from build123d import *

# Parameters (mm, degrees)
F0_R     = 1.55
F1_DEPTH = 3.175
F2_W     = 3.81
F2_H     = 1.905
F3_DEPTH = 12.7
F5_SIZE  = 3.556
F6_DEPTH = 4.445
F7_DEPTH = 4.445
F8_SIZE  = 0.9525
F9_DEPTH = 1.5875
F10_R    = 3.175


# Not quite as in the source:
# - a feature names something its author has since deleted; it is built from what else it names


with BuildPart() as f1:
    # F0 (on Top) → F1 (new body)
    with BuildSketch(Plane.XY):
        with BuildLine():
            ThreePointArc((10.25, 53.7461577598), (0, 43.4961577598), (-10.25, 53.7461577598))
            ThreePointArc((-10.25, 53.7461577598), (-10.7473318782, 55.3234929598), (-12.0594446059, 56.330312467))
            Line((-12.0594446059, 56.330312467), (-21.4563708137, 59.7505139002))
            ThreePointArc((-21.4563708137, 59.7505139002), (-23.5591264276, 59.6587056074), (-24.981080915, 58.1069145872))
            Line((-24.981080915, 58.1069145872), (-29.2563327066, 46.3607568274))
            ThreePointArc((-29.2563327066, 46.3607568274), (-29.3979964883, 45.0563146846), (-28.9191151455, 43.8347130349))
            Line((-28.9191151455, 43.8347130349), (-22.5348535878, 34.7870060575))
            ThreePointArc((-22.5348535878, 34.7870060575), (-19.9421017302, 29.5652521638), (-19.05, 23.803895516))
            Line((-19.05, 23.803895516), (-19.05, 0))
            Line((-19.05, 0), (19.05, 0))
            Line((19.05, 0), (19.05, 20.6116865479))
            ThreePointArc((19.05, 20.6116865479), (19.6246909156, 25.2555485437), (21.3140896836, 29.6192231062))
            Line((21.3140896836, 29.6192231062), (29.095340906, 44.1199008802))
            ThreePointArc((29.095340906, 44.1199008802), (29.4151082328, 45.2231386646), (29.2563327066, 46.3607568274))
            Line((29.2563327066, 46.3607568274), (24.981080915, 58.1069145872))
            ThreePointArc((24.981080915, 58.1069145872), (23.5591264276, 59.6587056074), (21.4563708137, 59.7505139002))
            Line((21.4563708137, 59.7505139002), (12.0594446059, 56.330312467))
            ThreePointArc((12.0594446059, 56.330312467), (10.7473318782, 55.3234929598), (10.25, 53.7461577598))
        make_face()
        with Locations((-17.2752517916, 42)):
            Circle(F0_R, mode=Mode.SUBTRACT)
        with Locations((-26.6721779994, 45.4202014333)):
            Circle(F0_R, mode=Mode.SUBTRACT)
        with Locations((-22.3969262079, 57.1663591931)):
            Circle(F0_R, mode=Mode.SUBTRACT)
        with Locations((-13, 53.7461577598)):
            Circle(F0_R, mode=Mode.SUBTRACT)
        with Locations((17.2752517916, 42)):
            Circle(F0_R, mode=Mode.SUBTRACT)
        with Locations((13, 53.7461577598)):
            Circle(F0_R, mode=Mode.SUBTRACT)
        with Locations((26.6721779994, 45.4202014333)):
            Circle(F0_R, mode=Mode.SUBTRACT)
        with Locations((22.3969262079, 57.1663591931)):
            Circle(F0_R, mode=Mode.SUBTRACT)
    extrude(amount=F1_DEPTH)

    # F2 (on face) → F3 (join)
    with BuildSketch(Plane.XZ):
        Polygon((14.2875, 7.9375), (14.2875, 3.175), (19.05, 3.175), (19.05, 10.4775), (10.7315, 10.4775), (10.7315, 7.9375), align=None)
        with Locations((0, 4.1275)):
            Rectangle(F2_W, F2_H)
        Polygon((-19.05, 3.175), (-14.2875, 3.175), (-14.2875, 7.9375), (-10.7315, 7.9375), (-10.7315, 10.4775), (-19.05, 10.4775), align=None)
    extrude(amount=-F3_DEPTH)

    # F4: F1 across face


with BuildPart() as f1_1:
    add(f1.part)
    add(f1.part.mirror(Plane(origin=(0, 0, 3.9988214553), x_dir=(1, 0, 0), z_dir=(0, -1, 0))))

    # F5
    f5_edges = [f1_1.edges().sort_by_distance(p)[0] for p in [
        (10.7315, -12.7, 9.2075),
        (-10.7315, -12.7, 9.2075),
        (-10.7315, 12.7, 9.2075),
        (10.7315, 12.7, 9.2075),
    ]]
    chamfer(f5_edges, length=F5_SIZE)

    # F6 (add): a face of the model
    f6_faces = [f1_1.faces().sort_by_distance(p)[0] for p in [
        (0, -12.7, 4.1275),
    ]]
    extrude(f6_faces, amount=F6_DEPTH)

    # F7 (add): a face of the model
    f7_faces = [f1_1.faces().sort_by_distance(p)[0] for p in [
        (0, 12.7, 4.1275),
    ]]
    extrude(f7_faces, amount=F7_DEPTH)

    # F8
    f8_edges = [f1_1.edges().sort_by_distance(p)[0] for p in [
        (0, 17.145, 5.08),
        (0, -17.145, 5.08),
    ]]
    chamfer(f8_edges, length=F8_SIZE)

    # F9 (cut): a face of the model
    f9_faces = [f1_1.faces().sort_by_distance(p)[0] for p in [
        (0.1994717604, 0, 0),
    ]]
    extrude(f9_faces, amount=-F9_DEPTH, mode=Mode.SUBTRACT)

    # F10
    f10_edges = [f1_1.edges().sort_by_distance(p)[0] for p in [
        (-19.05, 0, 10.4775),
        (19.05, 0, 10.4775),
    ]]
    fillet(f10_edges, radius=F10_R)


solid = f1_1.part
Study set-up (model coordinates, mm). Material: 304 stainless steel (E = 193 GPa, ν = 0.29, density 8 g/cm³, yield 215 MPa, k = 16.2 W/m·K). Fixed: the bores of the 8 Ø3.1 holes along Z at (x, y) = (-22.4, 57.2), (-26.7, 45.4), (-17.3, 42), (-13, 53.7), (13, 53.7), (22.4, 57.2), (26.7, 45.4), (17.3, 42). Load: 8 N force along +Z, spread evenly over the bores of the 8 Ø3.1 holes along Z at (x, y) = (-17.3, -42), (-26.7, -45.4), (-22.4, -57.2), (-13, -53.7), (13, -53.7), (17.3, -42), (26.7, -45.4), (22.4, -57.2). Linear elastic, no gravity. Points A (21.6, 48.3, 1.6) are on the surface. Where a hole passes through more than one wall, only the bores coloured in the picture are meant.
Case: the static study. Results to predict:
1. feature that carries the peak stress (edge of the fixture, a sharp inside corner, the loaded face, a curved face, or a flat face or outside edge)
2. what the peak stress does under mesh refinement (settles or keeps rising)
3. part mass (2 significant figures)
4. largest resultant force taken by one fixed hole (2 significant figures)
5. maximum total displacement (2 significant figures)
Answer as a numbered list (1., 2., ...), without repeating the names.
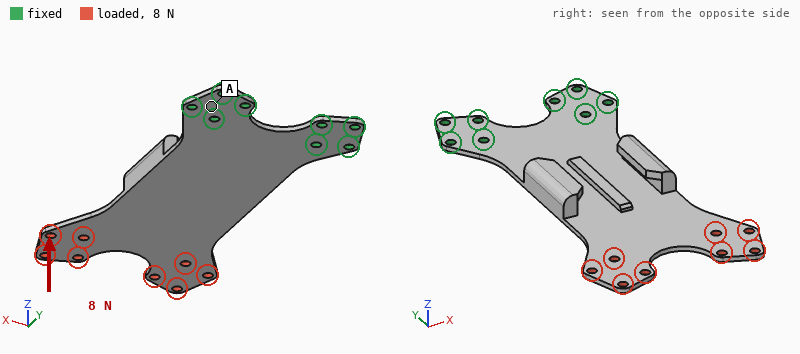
1. edge of the fixture
2. keeps rising
3. 77 g
4. 26 N
5. 0.71 mm
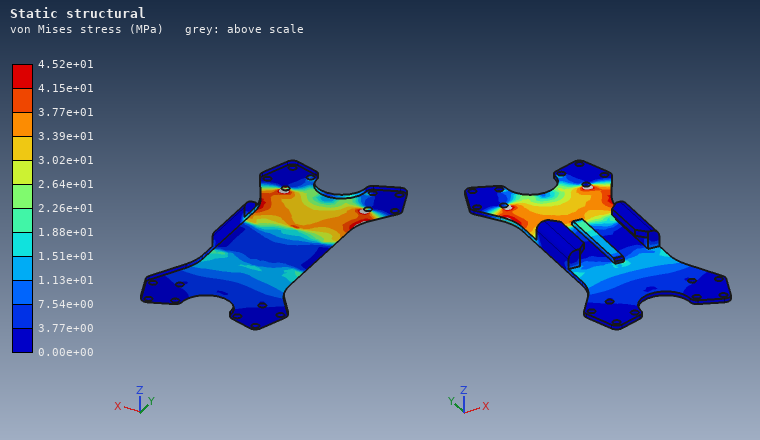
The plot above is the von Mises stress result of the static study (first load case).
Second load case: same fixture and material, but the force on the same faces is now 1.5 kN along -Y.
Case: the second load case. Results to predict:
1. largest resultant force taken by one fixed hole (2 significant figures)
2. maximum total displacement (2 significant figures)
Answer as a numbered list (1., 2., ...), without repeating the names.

1. 490 N
2. 61 µm
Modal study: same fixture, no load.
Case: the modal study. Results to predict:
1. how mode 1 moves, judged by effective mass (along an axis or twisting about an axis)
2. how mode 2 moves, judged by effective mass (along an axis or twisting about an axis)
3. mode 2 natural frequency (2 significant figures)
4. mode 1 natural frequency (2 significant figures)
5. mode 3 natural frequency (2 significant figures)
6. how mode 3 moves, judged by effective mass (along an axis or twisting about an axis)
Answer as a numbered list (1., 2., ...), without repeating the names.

1. along Z
2. twisting about Y
3. 580 Hz
4. 130 Hz
5. 880 Hz
6. along Z
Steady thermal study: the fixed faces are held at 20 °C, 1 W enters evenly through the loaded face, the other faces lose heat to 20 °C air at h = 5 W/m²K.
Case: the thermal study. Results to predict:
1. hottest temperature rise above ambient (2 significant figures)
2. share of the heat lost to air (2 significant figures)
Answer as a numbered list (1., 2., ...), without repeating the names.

1. 42 K
2. 76 %
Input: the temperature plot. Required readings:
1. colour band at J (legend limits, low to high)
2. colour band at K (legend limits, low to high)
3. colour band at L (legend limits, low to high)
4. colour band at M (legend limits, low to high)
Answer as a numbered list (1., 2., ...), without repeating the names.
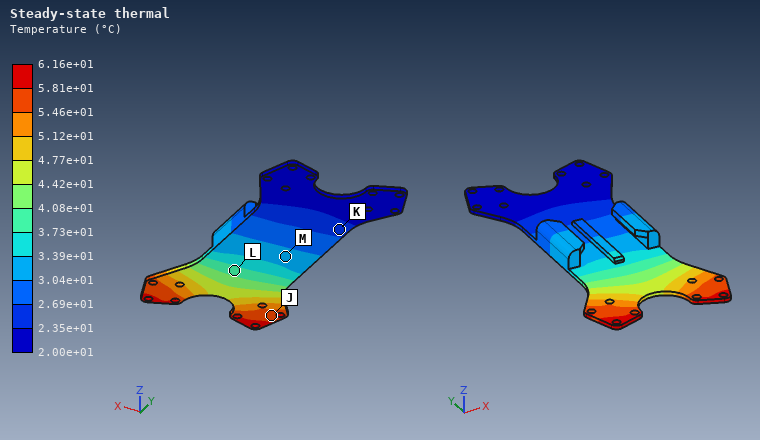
1. 5.46e+01 to 5.81e+01 °C
2. 2.35e+01 to 2.69e+01 °C
3. 3.73e+01 to 4.08e+01 °C
4. 3.04e+01 to 3.39e+01 °C
